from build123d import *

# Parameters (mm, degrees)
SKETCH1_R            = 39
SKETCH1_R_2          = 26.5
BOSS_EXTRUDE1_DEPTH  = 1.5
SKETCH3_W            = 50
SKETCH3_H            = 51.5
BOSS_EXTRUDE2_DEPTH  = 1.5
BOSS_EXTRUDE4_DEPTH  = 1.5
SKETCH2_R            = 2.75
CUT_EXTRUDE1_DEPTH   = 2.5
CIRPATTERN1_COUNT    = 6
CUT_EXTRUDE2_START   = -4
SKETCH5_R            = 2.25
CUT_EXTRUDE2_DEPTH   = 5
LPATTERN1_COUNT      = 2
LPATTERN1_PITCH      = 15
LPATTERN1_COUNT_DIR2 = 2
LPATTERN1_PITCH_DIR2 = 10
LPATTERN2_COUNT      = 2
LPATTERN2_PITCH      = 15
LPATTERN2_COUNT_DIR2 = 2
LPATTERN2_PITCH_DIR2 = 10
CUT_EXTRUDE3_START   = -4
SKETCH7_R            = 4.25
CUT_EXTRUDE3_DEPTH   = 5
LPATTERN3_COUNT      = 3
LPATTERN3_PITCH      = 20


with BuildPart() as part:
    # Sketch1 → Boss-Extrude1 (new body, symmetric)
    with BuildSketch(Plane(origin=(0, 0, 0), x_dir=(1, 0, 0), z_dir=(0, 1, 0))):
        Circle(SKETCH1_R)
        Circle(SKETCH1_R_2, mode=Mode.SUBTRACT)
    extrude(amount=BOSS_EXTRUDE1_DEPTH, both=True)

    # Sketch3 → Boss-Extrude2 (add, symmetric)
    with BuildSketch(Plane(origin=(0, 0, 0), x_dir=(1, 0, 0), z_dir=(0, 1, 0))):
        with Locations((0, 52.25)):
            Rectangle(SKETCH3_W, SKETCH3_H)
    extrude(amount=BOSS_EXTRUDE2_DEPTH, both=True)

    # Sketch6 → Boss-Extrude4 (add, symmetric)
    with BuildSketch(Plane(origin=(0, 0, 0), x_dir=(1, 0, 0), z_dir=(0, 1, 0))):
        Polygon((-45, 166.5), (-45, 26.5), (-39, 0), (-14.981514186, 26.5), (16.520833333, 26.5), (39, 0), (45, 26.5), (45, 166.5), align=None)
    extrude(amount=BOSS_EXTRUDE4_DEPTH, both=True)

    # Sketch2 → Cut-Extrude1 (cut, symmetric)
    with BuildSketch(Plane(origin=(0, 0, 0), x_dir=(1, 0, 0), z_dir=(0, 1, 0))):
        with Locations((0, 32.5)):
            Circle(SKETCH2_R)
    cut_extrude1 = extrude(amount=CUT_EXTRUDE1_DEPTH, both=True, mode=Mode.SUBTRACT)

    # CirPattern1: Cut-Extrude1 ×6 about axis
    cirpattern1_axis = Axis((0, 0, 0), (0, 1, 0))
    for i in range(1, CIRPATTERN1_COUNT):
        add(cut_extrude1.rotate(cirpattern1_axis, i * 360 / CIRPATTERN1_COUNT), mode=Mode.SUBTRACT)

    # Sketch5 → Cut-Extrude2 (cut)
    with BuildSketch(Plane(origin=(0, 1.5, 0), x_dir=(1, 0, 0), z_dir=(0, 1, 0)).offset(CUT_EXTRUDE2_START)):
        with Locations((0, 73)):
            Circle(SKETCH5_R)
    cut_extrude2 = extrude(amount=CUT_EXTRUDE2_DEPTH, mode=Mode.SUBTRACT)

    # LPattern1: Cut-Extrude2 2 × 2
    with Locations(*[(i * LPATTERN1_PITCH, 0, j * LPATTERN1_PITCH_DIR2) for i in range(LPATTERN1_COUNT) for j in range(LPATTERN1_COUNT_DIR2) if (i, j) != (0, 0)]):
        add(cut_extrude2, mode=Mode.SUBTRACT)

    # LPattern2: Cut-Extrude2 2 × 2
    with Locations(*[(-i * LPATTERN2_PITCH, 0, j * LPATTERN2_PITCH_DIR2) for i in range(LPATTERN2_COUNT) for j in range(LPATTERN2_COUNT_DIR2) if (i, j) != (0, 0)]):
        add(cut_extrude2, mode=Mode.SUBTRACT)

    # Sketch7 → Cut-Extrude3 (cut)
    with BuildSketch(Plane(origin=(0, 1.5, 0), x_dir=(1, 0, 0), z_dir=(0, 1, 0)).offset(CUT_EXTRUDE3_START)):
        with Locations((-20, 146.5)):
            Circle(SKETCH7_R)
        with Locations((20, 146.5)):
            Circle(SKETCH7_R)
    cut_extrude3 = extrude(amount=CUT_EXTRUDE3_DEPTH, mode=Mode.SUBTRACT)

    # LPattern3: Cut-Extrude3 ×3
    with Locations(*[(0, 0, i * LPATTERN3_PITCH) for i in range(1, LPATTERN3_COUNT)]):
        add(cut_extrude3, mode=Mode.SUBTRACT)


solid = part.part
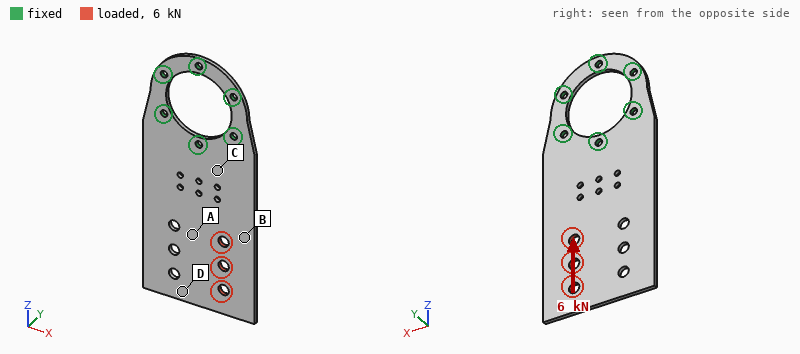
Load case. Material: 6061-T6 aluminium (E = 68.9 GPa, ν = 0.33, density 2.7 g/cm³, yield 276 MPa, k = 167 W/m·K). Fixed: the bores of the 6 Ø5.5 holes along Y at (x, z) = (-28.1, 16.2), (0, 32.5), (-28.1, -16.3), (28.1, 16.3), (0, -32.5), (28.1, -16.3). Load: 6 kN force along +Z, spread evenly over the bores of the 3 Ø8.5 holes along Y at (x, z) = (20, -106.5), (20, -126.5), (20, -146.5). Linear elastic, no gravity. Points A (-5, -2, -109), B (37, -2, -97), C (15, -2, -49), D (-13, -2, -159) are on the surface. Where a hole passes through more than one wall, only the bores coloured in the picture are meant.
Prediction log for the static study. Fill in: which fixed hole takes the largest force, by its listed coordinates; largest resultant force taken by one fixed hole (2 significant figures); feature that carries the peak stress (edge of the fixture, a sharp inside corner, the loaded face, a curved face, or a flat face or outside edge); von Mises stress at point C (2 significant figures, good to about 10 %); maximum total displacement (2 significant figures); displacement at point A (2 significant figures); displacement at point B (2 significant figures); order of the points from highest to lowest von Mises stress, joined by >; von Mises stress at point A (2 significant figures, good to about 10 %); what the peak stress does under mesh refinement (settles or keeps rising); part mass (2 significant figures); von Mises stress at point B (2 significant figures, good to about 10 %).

(28.1, -16.3)
3.3 kN
edge of the fixture
29 MPa
0.14 mm
0.055 mm
0.075 mm
B > C > A > D
17 MPa
keeps rising
120 g
44 MPa
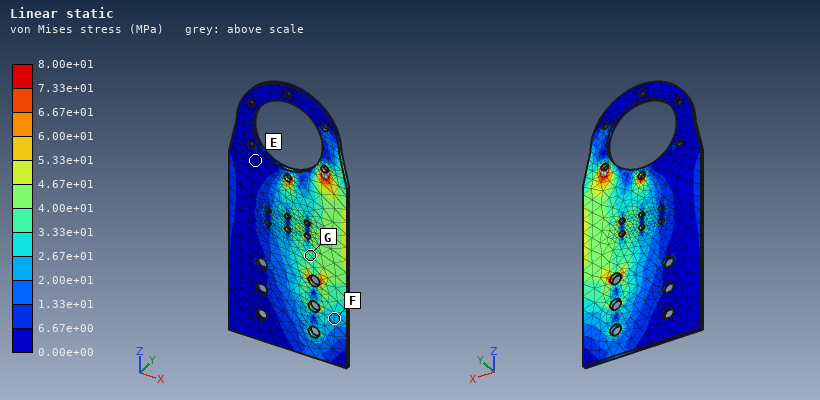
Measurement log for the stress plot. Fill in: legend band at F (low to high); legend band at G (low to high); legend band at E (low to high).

2.00e+01 to 2.67e+01 MPa
3.33e+01 to 4.00e+01 MPa
0.00e+00 to 6.67e+00 MPa
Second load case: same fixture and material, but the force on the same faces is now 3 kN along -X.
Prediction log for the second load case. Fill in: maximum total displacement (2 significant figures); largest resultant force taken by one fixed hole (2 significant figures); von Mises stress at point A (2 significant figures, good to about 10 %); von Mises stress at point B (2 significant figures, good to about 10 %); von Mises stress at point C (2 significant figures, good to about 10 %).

0.27 mm
3.8 kN
26 MPa
23 MPa
34 MPa
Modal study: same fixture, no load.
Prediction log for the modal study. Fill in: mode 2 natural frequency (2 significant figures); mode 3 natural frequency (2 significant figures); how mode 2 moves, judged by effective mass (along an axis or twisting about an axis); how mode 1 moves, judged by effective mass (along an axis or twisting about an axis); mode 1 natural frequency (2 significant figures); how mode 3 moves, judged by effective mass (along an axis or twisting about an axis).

400 Hz
770 Hz
twisting about Z
along Y
130 Hz
along Y
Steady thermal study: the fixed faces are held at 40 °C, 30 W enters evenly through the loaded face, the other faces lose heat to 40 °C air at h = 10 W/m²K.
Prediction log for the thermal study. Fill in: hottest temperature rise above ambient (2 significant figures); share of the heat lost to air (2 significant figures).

64 K
30 %
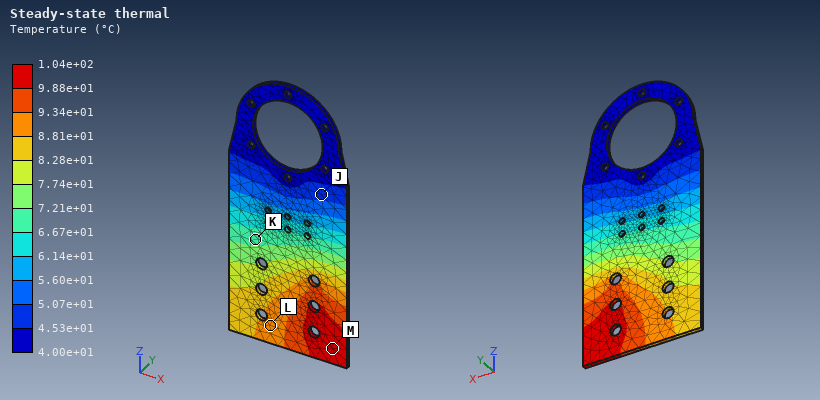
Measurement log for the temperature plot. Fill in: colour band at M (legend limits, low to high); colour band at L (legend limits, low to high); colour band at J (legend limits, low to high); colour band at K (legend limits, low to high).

9.88e+01 to 1.04e+02 °C
8.81e+01 to 9.34e+01 °C
4.53e+01 to 5.07e+01 °C
6.67e+01 to 7.21e+01 °C
